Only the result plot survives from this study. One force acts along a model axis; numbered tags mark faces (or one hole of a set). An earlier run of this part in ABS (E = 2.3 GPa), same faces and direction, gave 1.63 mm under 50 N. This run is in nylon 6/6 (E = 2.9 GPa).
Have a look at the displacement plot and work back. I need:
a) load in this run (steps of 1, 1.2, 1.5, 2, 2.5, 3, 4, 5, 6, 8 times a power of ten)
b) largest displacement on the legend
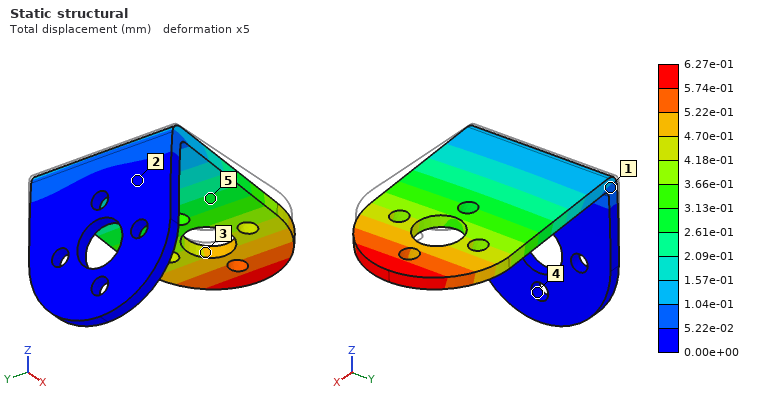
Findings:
25 N
6.27e-01 mm
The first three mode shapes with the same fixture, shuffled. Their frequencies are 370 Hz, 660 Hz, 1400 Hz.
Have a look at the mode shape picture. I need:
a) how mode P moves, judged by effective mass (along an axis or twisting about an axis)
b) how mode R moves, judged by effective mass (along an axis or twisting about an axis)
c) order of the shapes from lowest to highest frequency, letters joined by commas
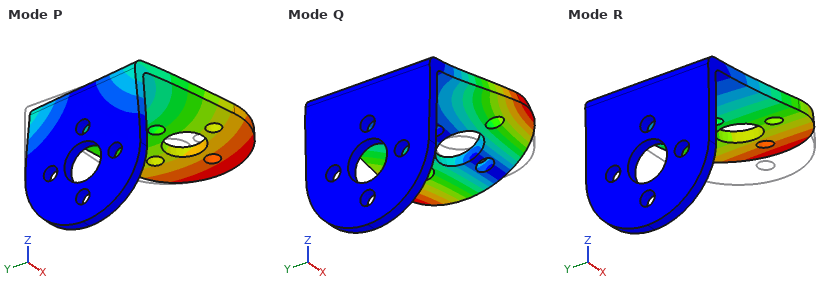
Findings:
along Y
along Z
R, P, Q
